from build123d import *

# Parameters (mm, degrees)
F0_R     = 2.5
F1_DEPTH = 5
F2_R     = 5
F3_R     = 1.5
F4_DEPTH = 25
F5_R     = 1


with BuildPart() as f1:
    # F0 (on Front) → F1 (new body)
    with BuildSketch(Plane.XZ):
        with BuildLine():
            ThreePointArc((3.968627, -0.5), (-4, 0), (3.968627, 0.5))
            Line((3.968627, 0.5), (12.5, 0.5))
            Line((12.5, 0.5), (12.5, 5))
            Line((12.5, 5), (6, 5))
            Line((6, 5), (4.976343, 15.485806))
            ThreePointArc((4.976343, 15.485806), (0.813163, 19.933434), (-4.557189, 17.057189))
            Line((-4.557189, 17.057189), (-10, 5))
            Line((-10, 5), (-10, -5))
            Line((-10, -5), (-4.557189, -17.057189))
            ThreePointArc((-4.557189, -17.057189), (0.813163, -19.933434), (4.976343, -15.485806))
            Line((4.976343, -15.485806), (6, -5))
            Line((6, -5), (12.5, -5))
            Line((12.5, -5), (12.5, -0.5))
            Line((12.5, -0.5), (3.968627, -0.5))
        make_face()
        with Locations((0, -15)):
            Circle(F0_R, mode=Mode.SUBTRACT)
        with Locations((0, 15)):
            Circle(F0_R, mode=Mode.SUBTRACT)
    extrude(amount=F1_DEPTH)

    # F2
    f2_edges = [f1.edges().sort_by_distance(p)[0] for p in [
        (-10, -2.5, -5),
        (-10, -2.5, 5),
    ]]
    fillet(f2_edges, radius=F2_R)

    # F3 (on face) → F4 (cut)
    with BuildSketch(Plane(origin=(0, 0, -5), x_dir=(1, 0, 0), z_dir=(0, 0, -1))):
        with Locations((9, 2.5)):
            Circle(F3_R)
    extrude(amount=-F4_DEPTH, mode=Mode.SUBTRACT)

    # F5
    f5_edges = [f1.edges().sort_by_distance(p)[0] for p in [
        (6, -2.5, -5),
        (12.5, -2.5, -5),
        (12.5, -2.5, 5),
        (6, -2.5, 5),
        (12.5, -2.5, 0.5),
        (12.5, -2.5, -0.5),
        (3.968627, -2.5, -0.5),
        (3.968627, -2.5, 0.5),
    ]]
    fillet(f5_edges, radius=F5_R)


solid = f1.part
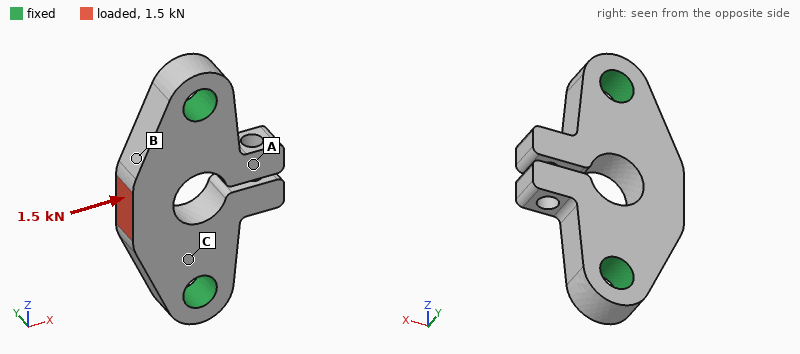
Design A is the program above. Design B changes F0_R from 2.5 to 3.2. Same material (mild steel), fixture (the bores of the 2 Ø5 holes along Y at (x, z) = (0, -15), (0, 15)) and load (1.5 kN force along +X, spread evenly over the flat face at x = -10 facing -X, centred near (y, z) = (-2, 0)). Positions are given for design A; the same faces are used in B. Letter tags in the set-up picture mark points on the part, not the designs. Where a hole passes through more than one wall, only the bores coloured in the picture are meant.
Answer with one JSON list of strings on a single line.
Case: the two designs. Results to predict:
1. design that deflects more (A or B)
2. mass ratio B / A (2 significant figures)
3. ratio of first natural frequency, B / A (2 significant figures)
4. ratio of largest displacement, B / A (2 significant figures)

["A", "0.95", "1.1", "0.90"]
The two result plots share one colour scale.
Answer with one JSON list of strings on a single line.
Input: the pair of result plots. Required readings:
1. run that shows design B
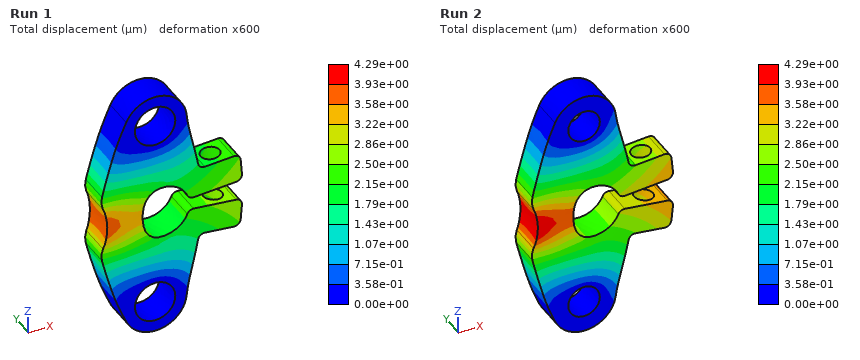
["Run 1"]
